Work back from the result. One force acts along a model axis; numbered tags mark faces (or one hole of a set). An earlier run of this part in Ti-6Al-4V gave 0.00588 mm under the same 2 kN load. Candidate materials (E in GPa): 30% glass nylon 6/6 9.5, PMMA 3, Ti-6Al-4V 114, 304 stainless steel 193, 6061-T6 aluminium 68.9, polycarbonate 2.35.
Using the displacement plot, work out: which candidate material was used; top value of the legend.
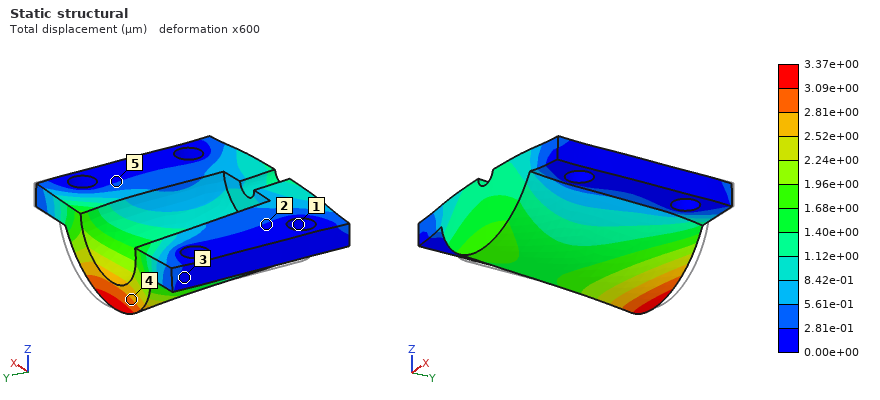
304 stainless steel
3.37e+00 µm
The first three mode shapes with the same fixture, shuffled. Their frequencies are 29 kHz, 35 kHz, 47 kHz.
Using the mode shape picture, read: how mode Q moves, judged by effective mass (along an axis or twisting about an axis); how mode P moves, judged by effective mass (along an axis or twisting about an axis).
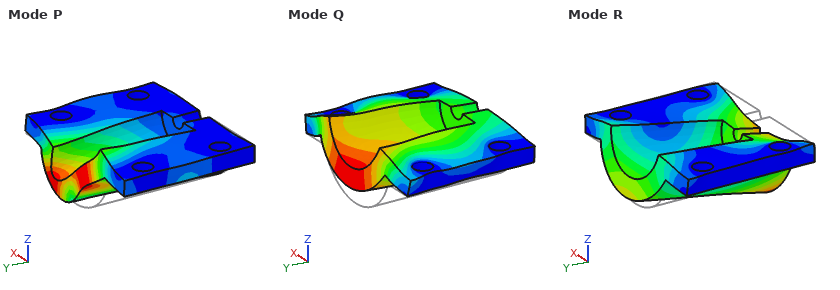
along Z
along X
